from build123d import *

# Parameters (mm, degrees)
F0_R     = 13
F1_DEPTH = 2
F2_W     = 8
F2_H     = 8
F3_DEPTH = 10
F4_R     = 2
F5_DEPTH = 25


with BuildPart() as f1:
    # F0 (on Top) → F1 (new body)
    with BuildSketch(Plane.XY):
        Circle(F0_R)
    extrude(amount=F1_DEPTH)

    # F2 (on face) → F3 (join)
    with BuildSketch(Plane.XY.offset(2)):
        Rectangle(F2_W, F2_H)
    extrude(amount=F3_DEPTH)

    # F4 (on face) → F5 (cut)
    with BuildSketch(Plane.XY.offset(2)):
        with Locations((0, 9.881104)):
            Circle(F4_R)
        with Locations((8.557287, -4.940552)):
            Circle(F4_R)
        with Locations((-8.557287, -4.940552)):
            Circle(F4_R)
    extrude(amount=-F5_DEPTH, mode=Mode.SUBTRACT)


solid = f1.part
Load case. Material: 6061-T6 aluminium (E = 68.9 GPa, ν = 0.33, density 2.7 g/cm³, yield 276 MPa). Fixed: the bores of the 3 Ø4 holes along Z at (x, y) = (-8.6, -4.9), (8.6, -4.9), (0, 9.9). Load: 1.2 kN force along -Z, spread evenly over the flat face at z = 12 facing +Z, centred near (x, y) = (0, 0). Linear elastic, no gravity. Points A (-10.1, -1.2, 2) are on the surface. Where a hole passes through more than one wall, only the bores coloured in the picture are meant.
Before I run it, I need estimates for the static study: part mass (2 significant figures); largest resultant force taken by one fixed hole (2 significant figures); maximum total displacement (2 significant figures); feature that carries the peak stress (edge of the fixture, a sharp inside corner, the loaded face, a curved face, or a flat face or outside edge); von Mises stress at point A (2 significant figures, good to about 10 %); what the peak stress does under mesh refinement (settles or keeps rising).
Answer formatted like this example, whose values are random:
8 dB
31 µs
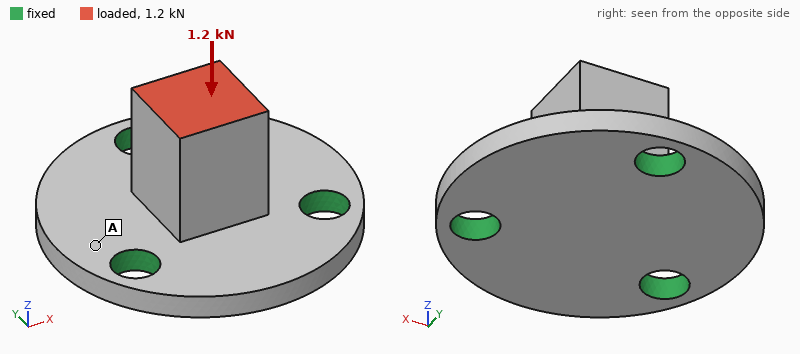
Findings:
4.4 g
410 N
18 µm
edge of the fixture
25 MPa
keeps rising
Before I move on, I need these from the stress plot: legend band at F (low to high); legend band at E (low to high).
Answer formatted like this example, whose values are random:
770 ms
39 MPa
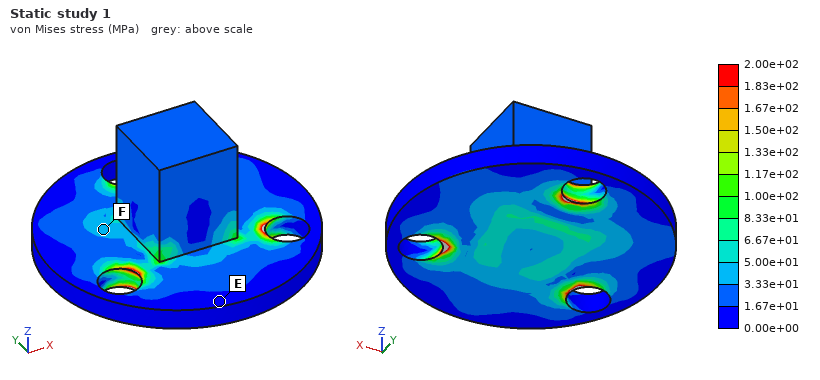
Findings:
3.33e+01 to 5.00e+01 MPa
0.00e+00 to 1.67e+01 MPa
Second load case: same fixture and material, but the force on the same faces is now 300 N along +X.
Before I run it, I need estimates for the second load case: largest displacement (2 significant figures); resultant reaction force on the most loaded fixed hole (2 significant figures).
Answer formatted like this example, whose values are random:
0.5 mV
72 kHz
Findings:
25 µm
260 N
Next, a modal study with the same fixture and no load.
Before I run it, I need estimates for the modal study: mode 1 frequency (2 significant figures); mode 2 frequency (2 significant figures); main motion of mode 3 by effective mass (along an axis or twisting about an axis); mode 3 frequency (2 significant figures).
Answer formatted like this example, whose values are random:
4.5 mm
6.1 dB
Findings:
21 kHz
21 kHz
along Z
27 kHz
